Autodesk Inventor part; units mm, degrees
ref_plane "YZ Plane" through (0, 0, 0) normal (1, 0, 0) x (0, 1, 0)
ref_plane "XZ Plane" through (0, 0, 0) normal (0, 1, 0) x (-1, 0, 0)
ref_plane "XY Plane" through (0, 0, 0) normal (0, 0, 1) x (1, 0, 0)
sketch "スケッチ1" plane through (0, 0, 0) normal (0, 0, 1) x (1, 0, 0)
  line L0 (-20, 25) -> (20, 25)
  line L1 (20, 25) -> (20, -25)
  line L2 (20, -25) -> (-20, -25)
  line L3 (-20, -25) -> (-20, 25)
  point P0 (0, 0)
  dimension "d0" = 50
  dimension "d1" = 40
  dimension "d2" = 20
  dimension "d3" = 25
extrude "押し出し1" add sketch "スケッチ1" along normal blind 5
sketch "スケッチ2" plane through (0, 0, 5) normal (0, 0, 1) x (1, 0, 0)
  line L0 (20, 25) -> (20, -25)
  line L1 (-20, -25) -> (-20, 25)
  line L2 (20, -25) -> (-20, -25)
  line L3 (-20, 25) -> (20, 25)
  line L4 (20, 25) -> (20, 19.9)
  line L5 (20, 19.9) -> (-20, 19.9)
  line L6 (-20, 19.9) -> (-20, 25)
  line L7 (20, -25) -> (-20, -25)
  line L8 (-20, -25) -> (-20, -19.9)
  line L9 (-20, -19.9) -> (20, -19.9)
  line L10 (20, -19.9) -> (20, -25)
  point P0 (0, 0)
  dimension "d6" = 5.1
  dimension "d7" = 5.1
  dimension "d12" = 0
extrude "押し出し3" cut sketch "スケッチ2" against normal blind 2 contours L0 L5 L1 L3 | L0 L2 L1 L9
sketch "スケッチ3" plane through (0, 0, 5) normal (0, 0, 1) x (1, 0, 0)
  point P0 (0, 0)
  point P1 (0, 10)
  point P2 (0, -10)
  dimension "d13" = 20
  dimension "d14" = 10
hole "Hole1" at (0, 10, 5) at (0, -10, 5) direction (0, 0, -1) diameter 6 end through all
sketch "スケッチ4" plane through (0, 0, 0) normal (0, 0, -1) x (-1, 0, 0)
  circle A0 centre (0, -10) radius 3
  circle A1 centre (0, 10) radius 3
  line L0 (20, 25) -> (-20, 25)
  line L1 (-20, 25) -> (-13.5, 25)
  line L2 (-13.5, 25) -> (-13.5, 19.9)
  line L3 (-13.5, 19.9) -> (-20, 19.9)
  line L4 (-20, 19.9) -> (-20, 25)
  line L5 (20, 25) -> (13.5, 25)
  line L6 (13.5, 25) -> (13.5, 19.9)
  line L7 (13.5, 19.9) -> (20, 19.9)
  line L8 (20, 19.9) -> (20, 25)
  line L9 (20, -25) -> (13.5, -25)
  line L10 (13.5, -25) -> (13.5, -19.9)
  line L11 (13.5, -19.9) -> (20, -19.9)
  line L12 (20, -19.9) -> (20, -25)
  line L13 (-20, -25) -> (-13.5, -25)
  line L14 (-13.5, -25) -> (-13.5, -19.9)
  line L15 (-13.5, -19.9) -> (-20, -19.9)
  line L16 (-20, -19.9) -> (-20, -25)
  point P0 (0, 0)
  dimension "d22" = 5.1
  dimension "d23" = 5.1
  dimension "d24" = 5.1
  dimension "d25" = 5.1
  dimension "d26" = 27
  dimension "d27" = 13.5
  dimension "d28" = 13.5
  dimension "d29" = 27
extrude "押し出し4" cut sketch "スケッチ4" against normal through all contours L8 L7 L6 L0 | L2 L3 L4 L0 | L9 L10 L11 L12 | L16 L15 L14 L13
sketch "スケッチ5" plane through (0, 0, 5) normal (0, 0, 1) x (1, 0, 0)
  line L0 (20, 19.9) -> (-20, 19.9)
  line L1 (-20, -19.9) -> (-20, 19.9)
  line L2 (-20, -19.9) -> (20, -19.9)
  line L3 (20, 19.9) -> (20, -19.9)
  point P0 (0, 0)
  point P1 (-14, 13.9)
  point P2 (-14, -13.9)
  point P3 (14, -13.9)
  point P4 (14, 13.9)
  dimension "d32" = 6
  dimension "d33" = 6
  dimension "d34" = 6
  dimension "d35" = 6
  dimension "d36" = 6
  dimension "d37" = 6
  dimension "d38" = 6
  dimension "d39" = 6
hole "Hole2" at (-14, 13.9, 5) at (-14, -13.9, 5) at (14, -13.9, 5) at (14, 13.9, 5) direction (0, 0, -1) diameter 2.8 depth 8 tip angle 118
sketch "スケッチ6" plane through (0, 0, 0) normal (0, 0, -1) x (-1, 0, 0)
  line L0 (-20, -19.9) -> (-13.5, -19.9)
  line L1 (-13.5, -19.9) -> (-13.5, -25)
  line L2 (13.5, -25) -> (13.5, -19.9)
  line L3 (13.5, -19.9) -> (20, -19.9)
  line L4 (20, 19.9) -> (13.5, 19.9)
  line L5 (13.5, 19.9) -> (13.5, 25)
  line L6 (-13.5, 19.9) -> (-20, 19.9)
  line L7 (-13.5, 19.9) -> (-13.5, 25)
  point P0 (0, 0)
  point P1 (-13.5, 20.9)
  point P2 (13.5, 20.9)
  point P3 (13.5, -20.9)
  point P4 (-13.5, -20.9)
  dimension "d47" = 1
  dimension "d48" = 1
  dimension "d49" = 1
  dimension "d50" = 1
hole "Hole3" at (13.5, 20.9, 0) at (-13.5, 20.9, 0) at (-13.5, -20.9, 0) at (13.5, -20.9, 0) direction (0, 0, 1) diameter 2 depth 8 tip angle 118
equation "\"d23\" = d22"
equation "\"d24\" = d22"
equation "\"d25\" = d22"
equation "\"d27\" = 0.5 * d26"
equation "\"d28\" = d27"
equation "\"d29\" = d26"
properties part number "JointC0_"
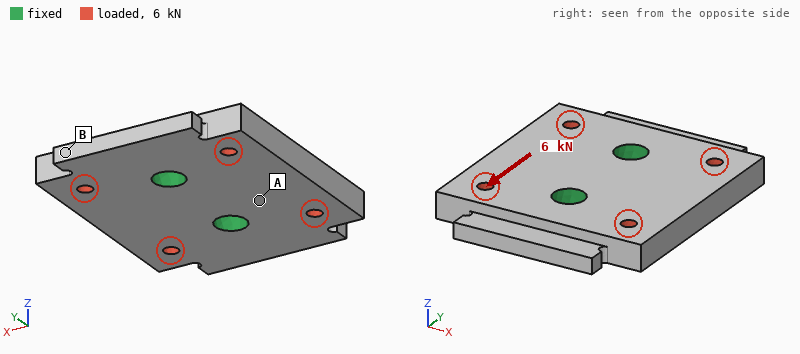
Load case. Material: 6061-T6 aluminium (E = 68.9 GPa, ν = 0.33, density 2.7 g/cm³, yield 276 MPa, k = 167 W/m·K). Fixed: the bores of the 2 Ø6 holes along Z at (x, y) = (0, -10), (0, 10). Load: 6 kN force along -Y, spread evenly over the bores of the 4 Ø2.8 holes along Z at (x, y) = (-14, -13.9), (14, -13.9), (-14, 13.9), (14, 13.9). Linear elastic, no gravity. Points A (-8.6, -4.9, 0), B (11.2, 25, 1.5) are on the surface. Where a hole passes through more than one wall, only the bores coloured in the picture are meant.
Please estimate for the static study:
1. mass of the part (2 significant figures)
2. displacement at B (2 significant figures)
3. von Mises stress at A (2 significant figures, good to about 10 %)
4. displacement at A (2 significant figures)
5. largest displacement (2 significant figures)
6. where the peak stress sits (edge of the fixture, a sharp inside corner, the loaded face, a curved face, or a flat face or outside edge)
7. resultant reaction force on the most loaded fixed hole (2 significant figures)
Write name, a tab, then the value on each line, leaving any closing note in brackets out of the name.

mass of the part	23 g
displacement at B	7.5 µm
von Mises stress at A	28 MPa
displacement at A	4.6 µm
largest displacement	11 µm
where the peak stress sits	the loaded face
resultant reaction force on the most loaded fixed hole	3.0 kN
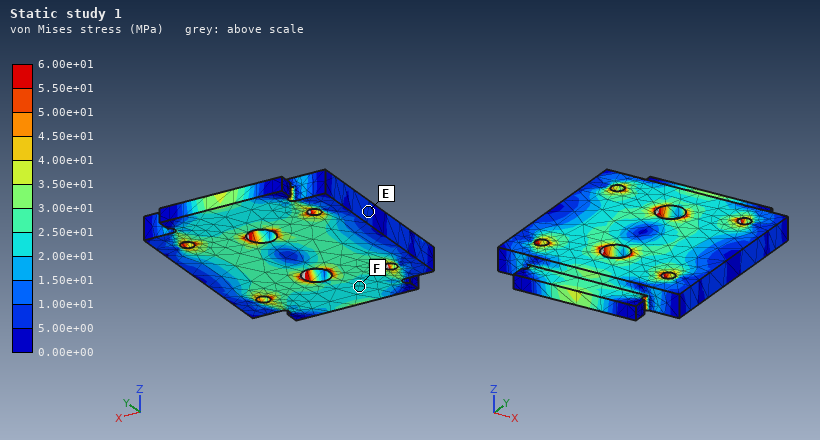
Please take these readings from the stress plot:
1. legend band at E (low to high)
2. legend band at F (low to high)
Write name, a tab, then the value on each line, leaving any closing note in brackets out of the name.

legend band at E	5.00e+00 to 1.00e+01 MPa
legend band at F	2.00e+01 to 2.50e+01 MPa
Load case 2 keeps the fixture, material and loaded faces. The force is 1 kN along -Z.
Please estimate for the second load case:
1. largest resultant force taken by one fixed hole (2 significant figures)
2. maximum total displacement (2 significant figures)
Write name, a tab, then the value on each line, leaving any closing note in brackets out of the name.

largest resultant force taken by one fixed hole	500 N
maximum total displacement	21 µm
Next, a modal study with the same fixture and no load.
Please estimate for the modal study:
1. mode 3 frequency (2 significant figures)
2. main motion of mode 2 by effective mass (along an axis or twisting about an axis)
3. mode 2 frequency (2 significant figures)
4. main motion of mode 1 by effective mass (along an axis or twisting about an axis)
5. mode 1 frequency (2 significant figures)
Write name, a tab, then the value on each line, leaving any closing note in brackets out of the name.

mode 3 frequency	14 kHz
main motion of mode 2 by effective mass	along Z
mode 2 frequency	12 kHz
main motion of mode 1 by effective mass	twisting about Y
mode 1 frequency	11 kHz
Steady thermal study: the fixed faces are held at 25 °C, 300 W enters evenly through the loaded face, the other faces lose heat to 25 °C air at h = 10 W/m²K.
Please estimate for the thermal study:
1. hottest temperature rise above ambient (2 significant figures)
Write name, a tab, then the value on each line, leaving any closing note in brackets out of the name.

hottest temperature rise above ambient	87 K
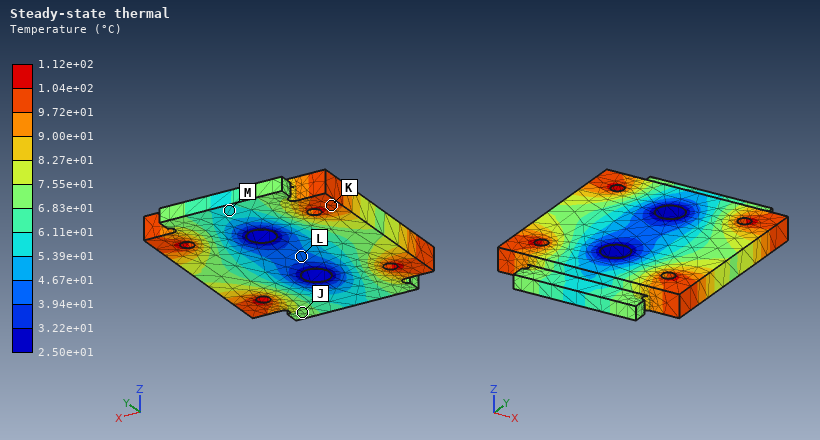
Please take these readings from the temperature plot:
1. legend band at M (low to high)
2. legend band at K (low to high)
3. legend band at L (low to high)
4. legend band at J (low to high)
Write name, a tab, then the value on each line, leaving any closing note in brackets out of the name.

legend band at M	5.39e+01 to 6.11e+01 °C
legend band at K	9.72e+01 to 1.04e+02 °C
legend band at L	3.94e+01 to 4.67e+01 °C
legend band at J	6.83e+01 to 7.55e+01 °C
